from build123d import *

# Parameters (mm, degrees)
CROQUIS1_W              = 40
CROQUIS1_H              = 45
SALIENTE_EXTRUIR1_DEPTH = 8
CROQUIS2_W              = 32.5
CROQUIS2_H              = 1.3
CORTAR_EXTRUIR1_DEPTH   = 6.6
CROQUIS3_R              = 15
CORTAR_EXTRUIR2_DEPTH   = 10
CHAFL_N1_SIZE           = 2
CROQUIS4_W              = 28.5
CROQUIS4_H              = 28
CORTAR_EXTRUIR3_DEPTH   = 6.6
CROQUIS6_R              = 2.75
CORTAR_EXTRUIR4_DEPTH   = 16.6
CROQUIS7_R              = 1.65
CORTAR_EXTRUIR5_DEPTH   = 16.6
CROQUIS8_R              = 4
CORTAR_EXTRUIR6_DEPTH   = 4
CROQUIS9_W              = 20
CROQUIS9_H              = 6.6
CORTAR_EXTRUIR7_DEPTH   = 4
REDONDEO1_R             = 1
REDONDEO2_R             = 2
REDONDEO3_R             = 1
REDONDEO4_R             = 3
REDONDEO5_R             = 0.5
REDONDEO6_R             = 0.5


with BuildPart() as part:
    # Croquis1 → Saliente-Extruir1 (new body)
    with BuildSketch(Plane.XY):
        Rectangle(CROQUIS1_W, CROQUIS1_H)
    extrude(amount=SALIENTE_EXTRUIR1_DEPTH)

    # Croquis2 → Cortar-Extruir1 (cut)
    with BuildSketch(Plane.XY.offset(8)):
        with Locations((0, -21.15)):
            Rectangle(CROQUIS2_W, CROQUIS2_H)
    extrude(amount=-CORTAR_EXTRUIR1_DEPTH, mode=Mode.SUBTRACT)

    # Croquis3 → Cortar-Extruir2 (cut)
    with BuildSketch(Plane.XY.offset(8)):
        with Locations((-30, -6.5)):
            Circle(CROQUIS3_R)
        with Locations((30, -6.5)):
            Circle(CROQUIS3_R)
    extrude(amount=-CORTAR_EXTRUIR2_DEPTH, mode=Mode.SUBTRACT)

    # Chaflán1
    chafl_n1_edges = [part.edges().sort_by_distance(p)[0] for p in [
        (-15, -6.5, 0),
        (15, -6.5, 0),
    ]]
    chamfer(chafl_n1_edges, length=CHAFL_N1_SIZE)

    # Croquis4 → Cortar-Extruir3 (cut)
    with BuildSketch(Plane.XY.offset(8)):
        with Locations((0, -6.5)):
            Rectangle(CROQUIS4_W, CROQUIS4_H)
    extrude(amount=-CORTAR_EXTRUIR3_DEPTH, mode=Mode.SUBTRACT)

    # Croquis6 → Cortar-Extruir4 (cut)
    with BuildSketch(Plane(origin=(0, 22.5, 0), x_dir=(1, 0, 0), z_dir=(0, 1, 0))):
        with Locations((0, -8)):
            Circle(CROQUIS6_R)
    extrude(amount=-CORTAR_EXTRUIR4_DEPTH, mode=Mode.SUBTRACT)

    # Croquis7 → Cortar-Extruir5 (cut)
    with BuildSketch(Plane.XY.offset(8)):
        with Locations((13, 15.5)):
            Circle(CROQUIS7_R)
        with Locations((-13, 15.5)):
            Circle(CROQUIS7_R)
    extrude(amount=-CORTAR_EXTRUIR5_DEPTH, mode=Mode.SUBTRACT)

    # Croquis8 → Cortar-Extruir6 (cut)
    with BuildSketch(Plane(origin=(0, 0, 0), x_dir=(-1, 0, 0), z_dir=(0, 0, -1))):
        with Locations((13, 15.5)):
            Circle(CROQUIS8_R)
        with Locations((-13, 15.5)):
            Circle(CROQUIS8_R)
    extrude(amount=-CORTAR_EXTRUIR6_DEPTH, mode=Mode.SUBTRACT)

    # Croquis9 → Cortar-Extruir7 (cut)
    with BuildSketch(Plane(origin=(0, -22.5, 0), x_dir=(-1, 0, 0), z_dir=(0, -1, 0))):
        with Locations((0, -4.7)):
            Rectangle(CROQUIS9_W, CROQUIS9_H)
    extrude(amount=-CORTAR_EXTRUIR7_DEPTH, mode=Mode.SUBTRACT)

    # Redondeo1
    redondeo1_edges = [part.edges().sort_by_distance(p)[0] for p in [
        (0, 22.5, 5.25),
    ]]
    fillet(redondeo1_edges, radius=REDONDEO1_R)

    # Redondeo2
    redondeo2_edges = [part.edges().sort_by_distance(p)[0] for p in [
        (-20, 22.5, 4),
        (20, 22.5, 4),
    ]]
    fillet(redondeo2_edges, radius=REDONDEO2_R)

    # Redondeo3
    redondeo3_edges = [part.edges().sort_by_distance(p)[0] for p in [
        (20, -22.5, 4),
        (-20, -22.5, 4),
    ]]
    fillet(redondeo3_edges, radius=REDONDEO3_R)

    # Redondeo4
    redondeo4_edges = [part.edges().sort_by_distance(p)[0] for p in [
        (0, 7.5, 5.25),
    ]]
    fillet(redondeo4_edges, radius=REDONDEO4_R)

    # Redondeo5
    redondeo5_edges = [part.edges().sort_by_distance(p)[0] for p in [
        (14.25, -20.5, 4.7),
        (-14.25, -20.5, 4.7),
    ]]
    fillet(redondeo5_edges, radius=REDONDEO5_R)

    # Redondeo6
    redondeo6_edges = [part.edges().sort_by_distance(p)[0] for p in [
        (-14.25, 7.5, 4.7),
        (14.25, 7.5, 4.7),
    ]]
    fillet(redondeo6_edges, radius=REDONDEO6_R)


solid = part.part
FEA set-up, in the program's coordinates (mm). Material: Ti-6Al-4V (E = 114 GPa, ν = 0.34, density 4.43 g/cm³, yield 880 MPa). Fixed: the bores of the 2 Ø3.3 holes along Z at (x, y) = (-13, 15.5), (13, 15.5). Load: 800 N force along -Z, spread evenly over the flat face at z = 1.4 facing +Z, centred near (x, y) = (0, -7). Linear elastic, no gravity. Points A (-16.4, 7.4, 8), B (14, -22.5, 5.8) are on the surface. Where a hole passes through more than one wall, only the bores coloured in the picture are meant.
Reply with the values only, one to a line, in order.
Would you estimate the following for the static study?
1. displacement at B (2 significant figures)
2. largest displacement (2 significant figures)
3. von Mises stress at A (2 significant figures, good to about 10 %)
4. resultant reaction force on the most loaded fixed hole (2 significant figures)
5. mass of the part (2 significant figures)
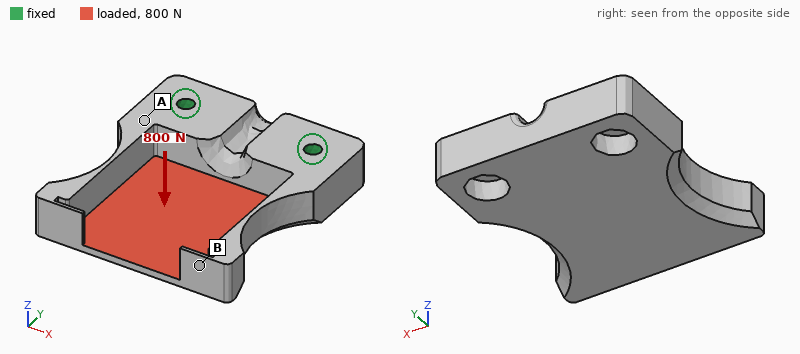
0.22 mm
0.37 mm
88 MPa
410 N
30 g
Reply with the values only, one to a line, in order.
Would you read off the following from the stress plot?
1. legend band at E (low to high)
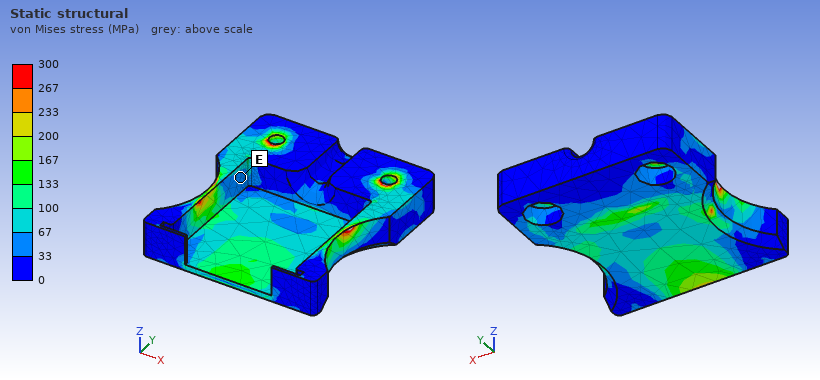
33 to 67 MPa
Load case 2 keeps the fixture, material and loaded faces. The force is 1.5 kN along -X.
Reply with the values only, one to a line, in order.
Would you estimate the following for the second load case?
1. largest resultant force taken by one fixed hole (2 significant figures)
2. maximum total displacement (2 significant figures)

1.4 kN
0.10 mm
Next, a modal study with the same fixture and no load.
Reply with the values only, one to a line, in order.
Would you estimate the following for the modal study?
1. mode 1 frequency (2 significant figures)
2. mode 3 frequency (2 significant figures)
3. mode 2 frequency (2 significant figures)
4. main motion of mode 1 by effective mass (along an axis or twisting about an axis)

3300 Hz
4500 Hz
3500 Hz
along Z
